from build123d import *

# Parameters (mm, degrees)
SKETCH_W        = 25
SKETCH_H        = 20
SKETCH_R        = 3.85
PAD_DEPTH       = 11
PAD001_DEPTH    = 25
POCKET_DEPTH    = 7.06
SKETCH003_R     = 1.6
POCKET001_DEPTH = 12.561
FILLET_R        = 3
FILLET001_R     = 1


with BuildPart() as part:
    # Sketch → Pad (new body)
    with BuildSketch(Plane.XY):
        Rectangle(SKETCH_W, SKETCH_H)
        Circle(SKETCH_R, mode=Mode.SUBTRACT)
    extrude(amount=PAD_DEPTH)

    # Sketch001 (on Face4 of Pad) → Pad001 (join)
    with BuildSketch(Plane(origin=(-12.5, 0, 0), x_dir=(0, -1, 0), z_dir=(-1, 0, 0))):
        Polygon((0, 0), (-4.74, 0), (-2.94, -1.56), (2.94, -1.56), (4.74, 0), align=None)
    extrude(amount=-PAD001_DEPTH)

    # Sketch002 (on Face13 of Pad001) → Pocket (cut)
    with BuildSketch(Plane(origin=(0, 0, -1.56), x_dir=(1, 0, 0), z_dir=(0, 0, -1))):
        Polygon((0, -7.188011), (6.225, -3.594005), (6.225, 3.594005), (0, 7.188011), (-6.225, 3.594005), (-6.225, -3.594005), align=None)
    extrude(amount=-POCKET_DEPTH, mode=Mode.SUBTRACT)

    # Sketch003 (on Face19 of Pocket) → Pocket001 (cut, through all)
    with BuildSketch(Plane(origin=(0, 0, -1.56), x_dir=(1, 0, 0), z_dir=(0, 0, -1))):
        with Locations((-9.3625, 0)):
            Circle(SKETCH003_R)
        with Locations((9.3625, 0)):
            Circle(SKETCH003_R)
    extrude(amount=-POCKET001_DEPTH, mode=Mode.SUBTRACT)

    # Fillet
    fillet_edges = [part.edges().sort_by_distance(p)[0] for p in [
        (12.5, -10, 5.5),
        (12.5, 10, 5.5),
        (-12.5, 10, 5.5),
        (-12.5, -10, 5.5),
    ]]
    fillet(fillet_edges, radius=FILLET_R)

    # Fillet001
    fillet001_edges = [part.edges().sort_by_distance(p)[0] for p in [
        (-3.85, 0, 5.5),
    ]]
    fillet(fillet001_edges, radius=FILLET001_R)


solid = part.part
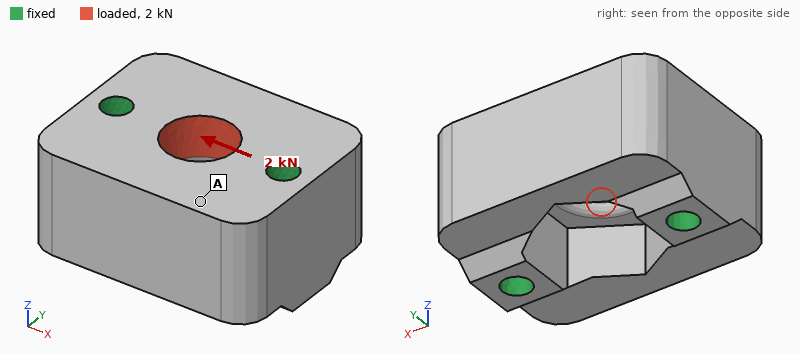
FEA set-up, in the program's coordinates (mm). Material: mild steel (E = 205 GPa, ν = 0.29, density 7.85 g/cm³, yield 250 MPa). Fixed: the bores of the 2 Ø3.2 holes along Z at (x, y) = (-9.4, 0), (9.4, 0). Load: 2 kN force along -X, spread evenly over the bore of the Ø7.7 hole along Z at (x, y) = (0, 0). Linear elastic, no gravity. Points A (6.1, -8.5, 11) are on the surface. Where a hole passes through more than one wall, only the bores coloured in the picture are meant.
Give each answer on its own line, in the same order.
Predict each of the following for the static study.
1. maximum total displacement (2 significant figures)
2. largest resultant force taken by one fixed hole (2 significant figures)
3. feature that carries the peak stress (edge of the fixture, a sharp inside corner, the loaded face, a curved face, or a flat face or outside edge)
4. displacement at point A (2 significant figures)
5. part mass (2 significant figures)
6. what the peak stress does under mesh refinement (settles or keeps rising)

0.85 µm
1.0 kN
edge of the fixture
0.50 µm
34 g
keeps rising
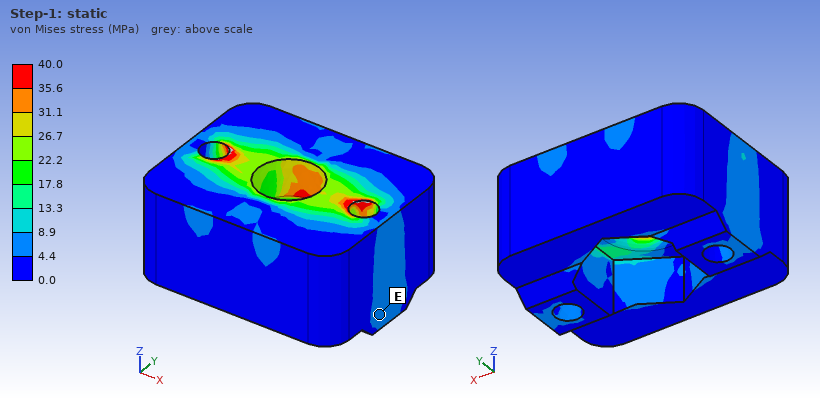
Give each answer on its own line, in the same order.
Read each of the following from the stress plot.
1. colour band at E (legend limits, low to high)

4.4 to 8.9 MPa
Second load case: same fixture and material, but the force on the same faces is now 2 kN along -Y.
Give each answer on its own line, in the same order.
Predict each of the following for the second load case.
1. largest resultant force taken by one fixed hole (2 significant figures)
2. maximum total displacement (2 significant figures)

1.0 kN
1.5 µm
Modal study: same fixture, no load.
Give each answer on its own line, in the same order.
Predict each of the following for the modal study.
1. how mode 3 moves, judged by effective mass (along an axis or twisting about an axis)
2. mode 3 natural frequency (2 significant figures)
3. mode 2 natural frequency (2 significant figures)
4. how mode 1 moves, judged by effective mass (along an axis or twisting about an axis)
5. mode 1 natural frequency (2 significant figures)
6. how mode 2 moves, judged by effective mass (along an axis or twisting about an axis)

twisting about Z
53 kHz
50 kHz
twisting about X
48 kHz
along Z
